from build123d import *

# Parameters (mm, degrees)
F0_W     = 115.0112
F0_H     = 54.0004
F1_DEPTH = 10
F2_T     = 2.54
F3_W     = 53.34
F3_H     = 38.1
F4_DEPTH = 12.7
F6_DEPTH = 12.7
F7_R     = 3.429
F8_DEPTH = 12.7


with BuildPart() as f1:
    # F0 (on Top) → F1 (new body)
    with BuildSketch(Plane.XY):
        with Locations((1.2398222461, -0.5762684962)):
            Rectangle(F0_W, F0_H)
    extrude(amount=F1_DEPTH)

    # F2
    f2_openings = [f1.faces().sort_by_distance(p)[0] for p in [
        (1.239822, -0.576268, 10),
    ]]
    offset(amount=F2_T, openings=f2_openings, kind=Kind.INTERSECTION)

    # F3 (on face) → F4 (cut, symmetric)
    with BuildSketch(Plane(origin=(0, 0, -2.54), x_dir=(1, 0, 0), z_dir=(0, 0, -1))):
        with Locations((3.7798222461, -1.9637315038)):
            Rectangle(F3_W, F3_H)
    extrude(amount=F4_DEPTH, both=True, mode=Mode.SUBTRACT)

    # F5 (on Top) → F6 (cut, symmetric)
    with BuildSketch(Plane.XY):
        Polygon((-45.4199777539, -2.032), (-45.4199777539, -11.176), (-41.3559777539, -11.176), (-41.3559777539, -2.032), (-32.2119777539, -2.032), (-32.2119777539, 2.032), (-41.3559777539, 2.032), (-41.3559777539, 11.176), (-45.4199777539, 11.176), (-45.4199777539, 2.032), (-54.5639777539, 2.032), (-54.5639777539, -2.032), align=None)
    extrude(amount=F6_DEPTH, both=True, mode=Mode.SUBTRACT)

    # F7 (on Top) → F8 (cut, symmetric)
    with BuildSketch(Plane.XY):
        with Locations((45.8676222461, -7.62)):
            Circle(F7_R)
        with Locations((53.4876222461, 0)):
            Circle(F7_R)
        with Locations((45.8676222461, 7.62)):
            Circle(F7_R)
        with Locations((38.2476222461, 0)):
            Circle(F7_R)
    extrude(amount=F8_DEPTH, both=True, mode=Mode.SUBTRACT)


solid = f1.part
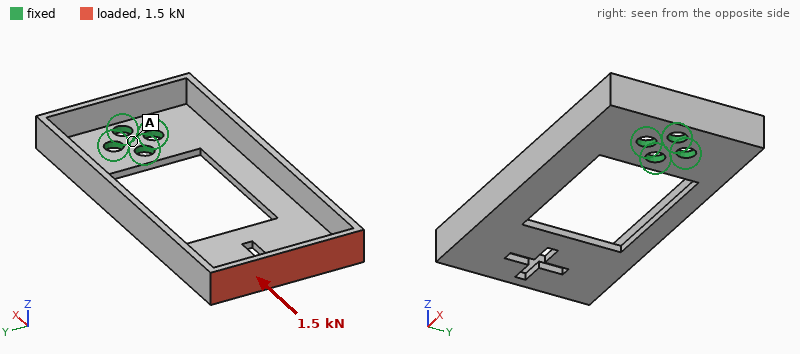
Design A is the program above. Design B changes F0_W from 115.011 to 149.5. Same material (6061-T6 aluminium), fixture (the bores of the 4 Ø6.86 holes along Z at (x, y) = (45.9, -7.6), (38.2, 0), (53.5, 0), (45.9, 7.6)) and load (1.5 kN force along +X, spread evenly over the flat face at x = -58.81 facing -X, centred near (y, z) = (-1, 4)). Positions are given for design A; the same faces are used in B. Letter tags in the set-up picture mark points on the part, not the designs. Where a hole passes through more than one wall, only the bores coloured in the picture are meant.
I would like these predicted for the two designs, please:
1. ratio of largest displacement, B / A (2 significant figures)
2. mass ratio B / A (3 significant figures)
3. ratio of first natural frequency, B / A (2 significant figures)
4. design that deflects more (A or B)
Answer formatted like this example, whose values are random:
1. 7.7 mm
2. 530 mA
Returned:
1. 1.2
2. 1.33
3. 0.75
4. B
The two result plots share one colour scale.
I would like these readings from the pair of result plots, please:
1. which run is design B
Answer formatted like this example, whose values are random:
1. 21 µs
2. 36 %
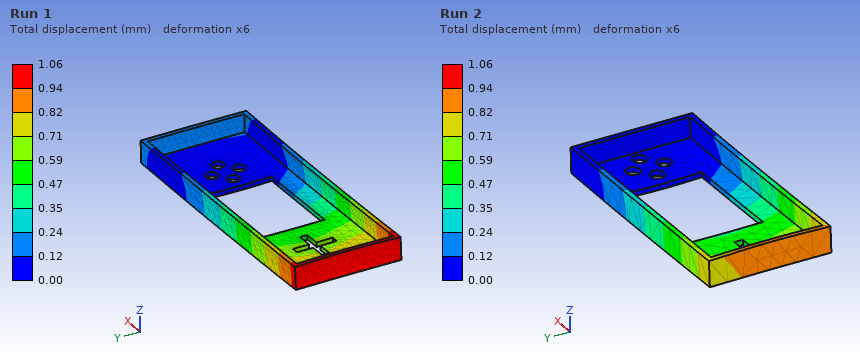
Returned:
1. Run 1
